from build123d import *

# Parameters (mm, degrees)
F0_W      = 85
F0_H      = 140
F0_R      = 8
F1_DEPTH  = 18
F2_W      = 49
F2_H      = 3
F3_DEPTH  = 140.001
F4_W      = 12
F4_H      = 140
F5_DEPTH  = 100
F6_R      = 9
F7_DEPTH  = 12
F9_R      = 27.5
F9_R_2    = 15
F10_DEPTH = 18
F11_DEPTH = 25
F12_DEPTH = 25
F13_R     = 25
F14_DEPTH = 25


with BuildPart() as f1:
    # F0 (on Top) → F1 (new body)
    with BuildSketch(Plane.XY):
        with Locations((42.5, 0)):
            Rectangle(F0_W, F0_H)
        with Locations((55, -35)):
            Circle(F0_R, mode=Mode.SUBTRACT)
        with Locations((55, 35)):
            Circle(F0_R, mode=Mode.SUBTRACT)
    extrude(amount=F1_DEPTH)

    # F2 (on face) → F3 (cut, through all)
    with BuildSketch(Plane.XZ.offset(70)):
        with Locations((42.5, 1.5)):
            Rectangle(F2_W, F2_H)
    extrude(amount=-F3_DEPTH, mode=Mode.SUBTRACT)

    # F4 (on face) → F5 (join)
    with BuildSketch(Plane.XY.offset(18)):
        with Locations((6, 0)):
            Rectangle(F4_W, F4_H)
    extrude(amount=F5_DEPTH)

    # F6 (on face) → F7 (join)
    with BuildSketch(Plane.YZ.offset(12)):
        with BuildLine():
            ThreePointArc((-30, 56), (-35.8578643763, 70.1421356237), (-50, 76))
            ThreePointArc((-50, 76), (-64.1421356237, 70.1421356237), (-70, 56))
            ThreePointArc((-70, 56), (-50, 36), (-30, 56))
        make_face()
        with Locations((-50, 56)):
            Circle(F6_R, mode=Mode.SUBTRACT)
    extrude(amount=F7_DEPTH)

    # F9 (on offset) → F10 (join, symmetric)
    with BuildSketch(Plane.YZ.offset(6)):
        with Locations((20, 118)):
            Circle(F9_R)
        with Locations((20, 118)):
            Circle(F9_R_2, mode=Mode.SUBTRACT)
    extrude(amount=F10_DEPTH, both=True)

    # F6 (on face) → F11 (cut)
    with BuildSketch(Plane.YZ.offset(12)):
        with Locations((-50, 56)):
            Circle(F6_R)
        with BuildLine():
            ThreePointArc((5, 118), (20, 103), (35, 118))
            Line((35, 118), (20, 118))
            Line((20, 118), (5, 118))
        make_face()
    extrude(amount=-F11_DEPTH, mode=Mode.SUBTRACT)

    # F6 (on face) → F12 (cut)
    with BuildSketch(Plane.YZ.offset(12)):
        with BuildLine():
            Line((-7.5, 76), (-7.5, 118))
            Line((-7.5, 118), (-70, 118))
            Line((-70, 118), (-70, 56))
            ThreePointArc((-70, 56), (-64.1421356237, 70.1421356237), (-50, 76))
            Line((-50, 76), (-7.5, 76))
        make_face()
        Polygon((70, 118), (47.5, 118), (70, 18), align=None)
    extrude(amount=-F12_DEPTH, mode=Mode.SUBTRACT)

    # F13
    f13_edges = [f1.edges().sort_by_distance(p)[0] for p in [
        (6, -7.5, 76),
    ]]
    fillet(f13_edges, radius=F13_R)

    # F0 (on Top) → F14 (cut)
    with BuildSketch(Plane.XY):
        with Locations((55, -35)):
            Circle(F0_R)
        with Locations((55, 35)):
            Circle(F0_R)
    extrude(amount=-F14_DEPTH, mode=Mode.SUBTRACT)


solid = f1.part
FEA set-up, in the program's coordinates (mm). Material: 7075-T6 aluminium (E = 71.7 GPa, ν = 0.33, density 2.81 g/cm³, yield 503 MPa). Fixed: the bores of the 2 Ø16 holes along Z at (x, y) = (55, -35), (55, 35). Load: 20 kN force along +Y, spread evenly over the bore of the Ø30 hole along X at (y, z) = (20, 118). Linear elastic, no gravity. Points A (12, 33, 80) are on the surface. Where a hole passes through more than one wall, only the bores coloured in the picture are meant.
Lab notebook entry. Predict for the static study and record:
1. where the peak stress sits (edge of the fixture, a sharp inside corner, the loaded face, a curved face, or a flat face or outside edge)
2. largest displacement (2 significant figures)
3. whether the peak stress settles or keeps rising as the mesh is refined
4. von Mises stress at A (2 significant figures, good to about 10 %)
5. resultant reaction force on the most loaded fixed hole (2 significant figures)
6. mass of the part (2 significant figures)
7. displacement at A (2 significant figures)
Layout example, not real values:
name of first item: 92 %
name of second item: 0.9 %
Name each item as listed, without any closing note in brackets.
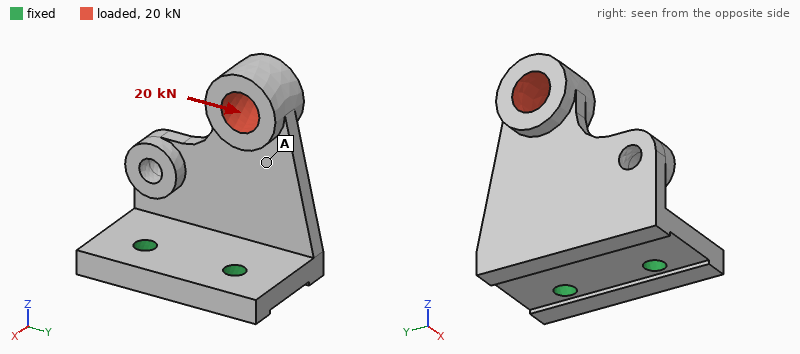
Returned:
where the peak stress sits: edge of the fixture
largest displacement: 1.5 mm
whether the peak stress settles or keeps rising as the mesh is refined: keeps rising
von Mises stress at A: 54 MPa
resultant reaction force on the most loaded fixed hole: 29 kN
mass of the part: 1.0 kg
displacement at A: 0.79 mm
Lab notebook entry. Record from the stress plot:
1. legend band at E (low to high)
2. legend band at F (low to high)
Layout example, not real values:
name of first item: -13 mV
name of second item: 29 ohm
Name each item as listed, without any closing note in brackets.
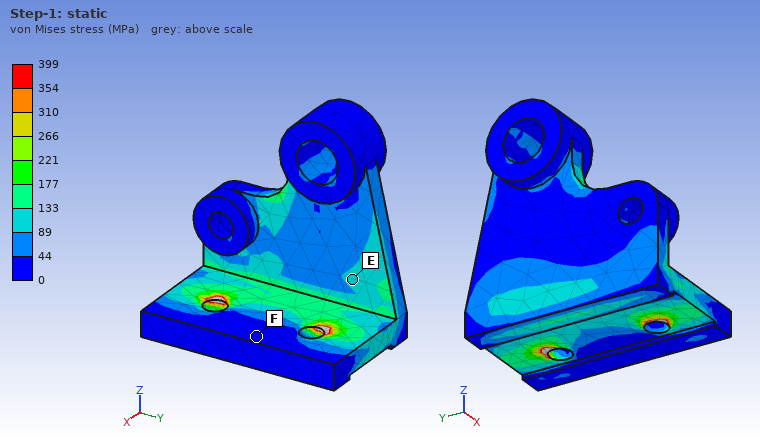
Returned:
legend band at E: 89 to 133 MPa
legend band at F: 0 to 44 MPa
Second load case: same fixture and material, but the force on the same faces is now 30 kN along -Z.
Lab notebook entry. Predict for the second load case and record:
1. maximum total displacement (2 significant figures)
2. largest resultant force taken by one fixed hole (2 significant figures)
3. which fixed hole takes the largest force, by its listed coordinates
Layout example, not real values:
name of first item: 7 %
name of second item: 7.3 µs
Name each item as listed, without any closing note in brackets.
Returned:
maximum total displacement: 1.8 mm
largest resultant force taken by one fixed hole: 22 kN
which fixed hole takes the largest force, by its listed coordinates: (55, 35)
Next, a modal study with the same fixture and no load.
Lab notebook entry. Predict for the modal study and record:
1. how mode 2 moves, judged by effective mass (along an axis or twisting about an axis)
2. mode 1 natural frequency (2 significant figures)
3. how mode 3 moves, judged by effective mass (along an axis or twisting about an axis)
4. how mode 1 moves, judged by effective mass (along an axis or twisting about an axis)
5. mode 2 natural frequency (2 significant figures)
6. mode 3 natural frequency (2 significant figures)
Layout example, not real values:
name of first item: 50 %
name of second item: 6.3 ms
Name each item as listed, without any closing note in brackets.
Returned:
how mode 2 moves, judged by effective mass: along Y
mode 1 natural frequency: 490 Hz
how mode 3 moves, judged by effective mass: along Z
how mode 1 moves, judged by effective mass: along X
mode 2 natural frequency: 1200 Hz
mode 3 natural frequency: 1800 Hz
